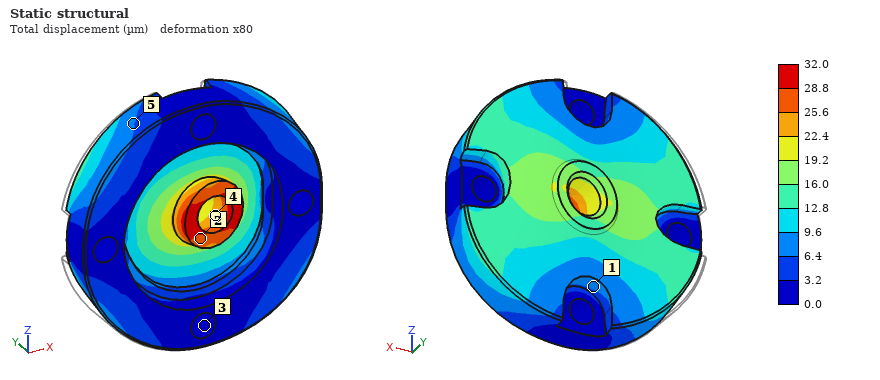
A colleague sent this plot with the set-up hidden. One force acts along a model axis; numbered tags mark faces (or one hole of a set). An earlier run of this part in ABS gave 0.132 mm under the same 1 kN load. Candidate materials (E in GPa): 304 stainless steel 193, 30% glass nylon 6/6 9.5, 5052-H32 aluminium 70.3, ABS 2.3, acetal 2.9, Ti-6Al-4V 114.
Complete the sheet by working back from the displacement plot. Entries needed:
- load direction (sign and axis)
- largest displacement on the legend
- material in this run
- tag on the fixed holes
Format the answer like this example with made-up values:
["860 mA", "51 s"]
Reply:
["+X", "32.0 µm", "30% glass nylon 6/6", "3"]
